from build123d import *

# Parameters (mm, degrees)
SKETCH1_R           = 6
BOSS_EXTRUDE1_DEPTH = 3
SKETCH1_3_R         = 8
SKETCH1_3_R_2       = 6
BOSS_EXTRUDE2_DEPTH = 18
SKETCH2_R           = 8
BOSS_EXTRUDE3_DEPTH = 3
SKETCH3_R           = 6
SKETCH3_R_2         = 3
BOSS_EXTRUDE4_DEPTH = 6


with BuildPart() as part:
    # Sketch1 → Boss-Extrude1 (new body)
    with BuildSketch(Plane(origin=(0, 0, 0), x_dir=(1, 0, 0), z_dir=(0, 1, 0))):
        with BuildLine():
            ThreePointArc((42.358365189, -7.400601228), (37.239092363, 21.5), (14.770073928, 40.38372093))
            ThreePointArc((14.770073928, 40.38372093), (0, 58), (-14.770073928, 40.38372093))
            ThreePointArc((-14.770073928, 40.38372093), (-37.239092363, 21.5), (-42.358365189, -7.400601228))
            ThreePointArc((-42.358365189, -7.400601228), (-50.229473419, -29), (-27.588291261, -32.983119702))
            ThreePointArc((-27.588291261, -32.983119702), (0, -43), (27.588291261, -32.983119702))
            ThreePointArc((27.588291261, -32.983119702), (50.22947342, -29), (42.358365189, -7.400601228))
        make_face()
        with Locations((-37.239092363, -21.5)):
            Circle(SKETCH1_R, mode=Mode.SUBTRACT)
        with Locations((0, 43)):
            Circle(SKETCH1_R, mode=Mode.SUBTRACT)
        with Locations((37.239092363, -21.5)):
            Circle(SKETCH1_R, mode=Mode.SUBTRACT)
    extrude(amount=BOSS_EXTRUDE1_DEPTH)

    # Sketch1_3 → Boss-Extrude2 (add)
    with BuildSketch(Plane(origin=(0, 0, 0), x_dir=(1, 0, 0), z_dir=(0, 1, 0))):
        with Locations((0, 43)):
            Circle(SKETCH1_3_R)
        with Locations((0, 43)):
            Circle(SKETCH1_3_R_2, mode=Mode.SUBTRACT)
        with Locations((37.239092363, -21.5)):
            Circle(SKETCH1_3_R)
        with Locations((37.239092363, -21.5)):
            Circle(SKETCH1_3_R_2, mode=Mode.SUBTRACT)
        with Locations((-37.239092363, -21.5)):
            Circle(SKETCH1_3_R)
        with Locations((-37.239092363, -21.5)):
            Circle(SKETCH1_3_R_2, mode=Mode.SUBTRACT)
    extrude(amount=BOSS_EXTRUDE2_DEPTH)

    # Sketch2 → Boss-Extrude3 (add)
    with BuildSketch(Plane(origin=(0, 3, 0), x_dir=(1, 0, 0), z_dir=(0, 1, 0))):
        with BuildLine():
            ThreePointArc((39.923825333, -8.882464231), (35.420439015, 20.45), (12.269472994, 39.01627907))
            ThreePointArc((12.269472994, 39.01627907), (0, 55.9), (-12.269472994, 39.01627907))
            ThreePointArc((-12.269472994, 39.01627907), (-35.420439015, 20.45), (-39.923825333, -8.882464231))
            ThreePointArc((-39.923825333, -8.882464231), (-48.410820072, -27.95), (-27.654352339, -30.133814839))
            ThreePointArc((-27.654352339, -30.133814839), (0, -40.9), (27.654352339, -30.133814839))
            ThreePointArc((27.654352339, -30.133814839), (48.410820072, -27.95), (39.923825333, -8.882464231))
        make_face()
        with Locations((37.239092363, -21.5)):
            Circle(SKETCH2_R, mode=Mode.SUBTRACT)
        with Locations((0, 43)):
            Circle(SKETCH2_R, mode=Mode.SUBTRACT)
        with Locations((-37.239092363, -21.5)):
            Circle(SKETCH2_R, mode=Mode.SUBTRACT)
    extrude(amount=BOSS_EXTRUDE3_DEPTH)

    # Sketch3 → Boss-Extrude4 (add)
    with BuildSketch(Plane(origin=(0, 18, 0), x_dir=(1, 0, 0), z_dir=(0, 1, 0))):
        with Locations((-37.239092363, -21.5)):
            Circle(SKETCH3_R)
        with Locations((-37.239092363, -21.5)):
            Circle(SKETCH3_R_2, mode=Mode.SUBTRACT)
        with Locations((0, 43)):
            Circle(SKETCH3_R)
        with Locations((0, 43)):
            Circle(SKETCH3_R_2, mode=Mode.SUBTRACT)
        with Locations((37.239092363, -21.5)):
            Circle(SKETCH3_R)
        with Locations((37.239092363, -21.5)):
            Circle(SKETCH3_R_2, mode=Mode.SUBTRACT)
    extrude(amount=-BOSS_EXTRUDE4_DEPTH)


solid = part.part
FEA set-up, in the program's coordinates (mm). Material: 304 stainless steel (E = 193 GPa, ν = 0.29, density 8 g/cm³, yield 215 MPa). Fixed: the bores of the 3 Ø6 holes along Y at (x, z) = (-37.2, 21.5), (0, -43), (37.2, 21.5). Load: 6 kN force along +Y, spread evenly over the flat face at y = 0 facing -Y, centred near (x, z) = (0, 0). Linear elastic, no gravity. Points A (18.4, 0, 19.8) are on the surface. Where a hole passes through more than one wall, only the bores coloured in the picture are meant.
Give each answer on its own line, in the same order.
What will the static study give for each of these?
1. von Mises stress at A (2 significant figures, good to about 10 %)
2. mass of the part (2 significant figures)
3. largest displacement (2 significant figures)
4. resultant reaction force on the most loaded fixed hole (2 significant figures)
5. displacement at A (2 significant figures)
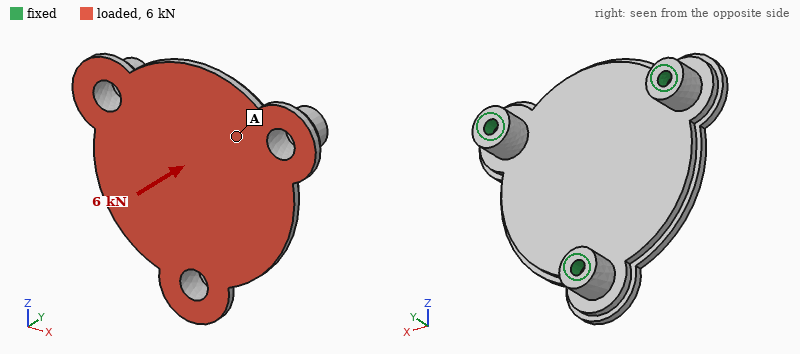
34 MPa
340 g
32 µm
2.2 kN
18 µm
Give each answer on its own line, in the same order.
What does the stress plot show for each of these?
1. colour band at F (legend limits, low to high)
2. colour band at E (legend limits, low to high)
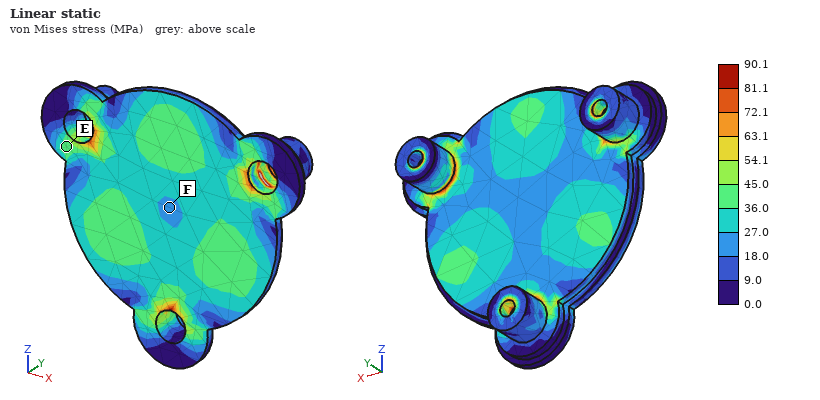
18.0 to 27.0 MPa
36.0 to 45.0 MPa
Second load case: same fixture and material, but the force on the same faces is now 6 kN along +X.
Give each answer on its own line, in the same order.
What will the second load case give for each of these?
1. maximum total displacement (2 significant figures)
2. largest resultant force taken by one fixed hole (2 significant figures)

21 µm
2.2 kN
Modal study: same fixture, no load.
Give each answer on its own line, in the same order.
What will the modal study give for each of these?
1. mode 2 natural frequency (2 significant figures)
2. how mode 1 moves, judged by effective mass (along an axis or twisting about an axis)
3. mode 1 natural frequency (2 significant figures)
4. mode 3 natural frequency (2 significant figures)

4700 Hz
along Y
4500 Hz
4700 Hz
